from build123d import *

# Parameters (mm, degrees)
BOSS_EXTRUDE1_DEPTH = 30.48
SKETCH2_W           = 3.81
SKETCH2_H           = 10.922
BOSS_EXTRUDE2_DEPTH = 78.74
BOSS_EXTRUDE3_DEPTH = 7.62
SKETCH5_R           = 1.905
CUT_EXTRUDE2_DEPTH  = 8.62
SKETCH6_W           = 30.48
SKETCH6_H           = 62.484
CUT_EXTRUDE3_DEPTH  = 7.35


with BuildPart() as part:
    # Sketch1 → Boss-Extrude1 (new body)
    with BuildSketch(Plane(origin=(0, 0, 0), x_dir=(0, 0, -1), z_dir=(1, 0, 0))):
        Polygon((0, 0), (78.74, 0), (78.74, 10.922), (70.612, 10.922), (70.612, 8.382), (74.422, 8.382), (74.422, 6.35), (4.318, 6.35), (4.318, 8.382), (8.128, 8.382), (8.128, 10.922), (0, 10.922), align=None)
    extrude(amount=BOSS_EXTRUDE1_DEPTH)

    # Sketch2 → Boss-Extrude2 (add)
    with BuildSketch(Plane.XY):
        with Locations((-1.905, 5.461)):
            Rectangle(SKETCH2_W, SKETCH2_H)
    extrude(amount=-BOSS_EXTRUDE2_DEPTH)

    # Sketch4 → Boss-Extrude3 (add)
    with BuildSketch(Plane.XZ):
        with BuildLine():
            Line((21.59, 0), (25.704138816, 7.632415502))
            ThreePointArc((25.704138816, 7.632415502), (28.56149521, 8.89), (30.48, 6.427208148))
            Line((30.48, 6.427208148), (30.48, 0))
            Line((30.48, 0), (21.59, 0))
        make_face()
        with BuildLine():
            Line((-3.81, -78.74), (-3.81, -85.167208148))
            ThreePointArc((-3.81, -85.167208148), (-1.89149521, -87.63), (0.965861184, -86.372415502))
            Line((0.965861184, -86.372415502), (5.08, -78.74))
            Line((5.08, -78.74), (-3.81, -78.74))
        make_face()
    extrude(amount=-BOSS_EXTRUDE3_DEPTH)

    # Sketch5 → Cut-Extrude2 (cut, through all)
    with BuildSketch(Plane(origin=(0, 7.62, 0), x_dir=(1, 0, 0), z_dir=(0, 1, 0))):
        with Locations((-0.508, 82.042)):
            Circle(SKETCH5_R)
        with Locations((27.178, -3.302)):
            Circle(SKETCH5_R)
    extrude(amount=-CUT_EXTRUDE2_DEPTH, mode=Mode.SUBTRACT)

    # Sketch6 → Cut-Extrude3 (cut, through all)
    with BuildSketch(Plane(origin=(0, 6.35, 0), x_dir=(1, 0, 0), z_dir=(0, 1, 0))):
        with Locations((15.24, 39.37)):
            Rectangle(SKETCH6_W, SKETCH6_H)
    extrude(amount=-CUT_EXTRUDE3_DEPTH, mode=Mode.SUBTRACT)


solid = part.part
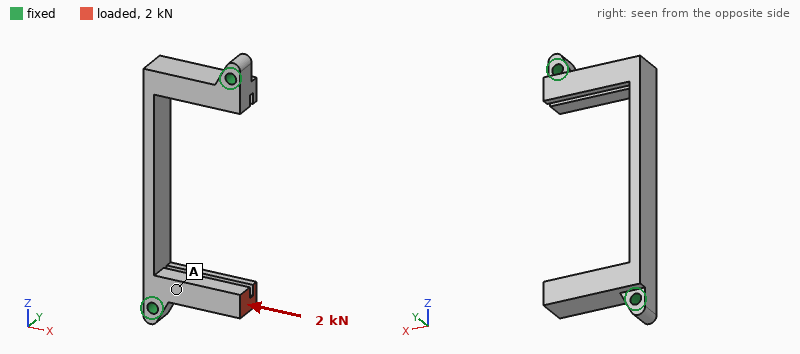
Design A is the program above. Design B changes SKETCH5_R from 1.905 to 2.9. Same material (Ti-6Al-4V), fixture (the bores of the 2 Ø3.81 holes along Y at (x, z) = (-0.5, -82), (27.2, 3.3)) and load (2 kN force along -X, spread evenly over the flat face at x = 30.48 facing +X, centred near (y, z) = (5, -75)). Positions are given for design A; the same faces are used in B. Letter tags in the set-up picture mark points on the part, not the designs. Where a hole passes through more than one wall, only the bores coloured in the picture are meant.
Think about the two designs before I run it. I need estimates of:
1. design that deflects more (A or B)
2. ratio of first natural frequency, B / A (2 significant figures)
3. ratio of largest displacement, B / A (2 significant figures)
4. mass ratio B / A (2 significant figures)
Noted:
A
1.1
0.63
0.97
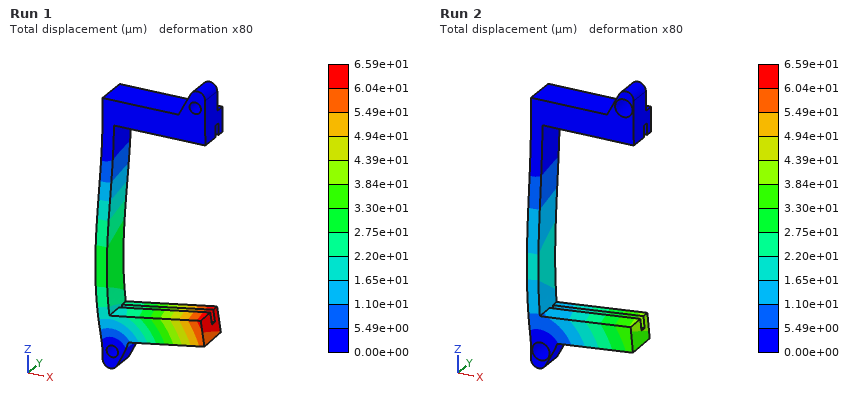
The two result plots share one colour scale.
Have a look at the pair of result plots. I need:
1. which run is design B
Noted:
Run 2
